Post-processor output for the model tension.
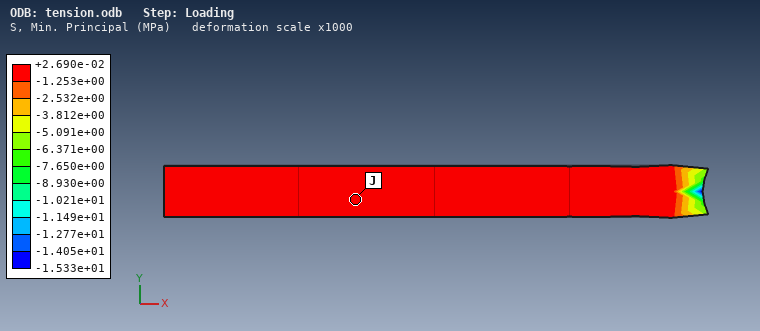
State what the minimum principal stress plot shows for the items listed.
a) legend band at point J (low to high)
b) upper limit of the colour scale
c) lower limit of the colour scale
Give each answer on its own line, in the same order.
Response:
-1.253e+00 to +2.690e-02 MPa
+2.690e-02 MPa
-1.533e+01 MPa
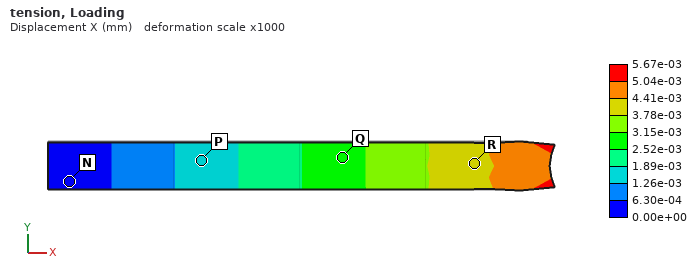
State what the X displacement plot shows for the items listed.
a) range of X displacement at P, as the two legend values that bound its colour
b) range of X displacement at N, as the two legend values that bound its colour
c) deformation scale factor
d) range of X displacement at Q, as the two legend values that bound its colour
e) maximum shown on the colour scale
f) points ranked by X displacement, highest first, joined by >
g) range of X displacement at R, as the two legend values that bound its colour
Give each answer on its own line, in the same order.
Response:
1.26e-03 to 1.89e-03 mm
0.00e+00 to 6.30e-04 mm
1000
2.52e-03 to 3.15e-03 mm
5.67e-03 mm
R > Q > P > N
3.78e-03 to 4.41e-03 mm
